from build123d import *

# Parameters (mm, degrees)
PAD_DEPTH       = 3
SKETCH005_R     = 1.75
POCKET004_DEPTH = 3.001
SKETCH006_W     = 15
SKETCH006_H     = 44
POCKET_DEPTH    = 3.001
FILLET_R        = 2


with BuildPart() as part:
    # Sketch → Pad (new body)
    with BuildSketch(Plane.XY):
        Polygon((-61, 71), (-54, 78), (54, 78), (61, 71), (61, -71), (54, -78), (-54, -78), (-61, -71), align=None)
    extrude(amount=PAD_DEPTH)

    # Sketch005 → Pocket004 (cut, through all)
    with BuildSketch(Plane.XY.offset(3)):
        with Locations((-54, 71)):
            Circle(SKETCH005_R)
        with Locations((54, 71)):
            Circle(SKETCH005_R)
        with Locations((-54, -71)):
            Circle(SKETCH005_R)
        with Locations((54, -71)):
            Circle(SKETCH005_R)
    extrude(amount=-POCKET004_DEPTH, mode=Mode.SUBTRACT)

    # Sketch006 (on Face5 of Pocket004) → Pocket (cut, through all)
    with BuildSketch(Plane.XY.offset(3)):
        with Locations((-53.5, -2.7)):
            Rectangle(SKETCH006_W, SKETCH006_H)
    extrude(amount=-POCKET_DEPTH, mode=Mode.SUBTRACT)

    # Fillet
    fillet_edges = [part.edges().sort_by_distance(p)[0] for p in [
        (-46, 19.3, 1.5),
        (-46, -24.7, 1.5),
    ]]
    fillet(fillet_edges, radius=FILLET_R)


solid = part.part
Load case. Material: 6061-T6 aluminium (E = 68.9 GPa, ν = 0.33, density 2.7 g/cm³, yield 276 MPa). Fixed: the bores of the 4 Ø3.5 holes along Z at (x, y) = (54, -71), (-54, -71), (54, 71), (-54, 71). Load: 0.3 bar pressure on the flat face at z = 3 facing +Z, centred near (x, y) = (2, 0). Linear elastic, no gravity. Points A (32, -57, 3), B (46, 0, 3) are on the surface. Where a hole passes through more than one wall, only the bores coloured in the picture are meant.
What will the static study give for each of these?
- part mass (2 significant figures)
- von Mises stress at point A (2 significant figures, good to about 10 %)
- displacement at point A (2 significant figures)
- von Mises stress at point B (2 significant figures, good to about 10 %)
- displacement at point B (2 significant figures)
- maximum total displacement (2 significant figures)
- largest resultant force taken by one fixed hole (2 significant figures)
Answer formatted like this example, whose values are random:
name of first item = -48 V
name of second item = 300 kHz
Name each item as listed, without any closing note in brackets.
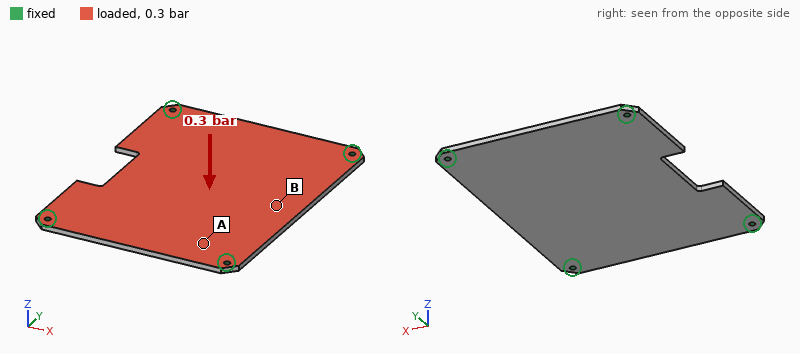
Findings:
part mass = 150 g
von Mises stress at point A = 8.3 MPa
displacement at point A = 0.13 mm
von Mises stress at point B = 23 MPa
displacement at point B = 0.35 mm
maximum total displacement = 0.42 mm
largest resultant force taken by one fixed hole = 140 N
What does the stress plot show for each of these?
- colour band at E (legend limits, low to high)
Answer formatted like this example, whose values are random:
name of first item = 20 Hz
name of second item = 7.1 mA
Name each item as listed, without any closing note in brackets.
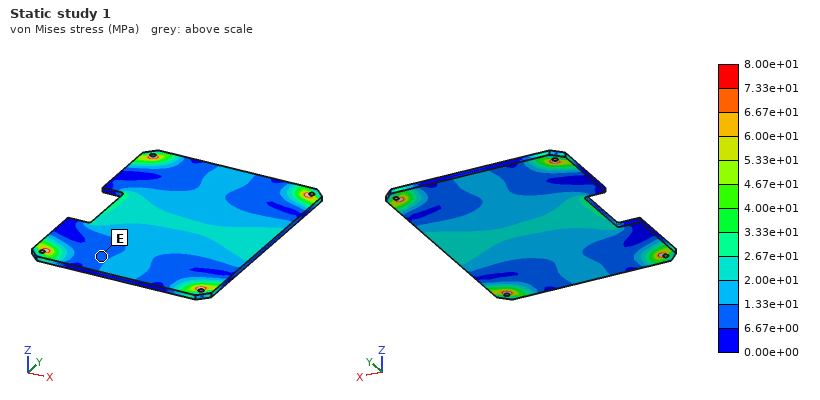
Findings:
colour band at E = 6.67e+00 to 1.33e+01 MPa
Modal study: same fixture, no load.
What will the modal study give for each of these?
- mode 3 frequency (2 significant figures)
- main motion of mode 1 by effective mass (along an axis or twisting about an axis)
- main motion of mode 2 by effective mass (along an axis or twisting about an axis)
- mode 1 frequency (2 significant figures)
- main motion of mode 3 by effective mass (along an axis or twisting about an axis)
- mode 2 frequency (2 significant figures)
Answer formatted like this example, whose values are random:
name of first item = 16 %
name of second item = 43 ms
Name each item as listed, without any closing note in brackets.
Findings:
mode 3 frequency = 1200 Hz
main motion of mode 1 by effective mass = along Z
main motion of mode 2 by effective mass = twisting about Y
mode 1 frequency = 560 Hz
main motion of mode 3 by effective mass = twisting about X
mode 2 frequency = 980 Hz
